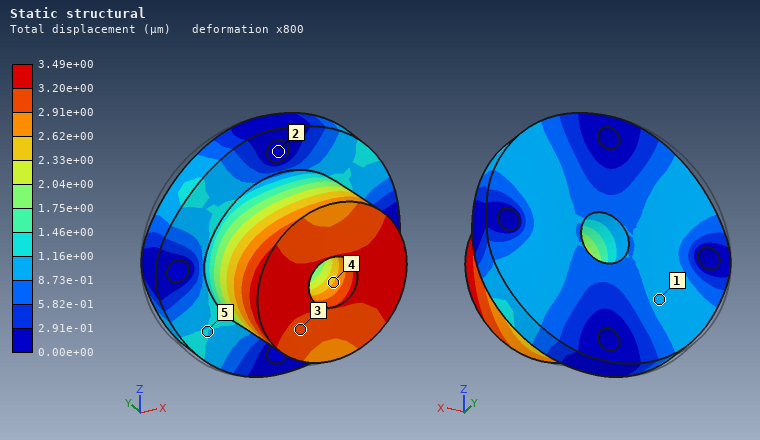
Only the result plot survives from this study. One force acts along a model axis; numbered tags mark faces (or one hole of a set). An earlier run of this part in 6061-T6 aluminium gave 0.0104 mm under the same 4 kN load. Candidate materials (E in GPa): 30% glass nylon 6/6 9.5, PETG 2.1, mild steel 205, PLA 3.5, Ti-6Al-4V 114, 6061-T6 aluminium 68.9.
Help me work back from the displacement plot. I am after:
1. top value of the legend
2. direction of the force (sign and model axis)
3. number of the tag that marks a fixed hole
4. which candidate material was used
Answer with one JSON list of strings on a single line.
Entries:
["3.49e+00 µm", "+X", "2", "mild steel"]
